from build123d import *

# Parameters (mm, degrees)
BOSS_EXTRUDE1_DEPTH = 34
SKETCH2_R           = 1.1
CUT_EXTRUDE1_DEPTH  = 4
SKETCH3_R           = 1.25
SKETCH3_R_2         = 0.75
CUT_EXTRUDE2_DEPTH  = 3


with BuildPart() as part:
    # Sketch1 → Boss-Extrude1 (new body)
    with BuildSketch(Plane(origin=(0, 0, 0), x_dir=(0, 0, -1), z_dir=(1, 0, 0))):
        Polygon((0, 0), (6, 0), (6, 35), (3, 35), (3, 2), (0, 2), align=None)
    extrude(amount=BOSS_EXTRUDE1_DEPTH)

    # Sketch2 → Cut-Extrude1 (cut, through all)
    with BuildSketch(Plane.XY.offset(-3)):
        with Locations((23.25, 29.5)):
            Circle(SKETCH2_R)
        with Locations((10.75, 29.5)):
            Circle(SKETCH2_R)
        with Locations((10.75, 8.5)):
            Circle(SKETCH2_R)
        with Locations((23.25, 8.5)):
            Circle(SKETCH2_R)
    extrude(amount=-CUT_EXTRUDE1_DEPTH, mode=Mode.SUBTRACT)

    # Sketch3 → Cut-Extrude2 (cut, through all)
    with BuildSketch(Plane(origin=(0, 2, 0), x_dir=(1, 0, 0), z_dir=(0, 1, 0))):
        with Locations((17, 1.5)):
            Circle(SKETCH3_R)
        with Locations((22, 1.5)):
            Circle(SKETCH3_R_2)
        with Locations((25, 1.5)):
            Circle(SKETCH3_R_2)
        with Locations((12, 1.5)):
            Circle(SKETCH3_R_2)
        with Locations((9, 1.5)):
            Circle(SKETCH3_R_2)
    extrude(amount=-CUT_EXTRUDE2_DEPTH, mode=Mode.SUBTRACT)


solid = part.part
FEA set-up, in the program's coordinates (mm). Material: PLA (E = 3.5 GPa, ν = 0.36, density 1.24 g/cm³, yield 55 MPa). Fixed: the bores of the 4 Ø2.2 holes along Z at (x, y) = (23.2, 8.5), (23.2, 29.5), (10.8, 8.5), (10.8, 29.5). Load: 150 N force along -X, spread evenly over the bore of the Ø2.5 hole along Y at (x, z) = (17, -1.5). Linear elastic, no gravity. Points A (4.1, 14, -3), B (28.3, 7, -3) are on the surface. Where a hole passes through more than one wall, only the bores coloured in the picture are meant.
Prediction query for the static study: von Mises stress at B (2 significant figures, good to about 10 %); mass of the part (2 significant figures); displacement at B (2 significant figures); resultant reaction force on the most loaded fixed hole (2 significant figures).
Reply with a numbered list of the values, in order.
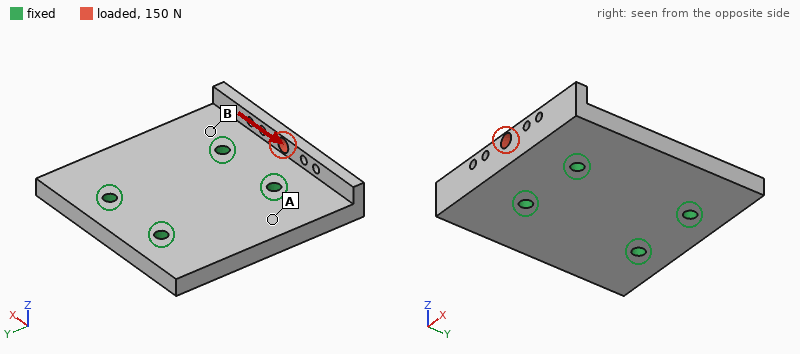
1. 3.6 MPa
2. 4.6 g
3. 15 µm
4. 98 N
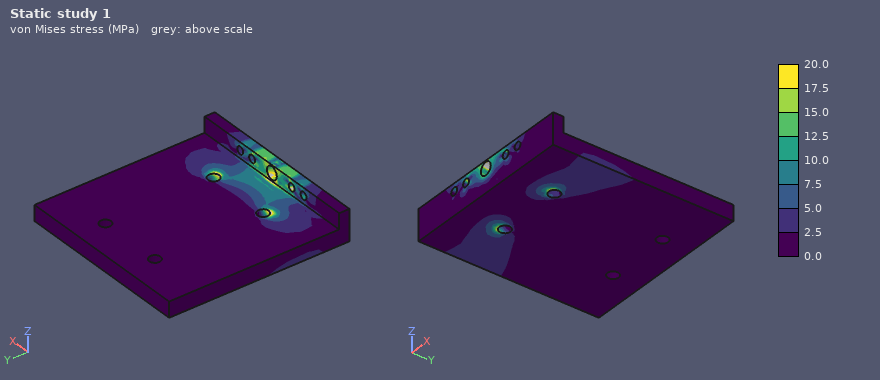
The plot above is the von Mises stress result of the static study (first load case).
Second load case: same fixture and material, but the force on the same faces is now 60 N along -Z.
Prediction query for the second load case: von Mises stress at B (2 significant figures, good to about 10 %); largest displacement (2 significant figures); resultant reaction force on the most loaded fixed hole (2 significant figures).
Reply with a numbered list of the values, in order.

1. 3.3 MPa
2. 0.11 mm
3. 33 N
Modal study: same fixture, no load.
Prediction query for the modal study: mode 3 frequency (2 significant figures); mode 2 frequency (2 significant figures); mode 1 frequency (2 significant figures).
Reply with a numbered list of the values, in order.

1. 6000 Hz
2. 5700 Hz
3. 5600 Hz
